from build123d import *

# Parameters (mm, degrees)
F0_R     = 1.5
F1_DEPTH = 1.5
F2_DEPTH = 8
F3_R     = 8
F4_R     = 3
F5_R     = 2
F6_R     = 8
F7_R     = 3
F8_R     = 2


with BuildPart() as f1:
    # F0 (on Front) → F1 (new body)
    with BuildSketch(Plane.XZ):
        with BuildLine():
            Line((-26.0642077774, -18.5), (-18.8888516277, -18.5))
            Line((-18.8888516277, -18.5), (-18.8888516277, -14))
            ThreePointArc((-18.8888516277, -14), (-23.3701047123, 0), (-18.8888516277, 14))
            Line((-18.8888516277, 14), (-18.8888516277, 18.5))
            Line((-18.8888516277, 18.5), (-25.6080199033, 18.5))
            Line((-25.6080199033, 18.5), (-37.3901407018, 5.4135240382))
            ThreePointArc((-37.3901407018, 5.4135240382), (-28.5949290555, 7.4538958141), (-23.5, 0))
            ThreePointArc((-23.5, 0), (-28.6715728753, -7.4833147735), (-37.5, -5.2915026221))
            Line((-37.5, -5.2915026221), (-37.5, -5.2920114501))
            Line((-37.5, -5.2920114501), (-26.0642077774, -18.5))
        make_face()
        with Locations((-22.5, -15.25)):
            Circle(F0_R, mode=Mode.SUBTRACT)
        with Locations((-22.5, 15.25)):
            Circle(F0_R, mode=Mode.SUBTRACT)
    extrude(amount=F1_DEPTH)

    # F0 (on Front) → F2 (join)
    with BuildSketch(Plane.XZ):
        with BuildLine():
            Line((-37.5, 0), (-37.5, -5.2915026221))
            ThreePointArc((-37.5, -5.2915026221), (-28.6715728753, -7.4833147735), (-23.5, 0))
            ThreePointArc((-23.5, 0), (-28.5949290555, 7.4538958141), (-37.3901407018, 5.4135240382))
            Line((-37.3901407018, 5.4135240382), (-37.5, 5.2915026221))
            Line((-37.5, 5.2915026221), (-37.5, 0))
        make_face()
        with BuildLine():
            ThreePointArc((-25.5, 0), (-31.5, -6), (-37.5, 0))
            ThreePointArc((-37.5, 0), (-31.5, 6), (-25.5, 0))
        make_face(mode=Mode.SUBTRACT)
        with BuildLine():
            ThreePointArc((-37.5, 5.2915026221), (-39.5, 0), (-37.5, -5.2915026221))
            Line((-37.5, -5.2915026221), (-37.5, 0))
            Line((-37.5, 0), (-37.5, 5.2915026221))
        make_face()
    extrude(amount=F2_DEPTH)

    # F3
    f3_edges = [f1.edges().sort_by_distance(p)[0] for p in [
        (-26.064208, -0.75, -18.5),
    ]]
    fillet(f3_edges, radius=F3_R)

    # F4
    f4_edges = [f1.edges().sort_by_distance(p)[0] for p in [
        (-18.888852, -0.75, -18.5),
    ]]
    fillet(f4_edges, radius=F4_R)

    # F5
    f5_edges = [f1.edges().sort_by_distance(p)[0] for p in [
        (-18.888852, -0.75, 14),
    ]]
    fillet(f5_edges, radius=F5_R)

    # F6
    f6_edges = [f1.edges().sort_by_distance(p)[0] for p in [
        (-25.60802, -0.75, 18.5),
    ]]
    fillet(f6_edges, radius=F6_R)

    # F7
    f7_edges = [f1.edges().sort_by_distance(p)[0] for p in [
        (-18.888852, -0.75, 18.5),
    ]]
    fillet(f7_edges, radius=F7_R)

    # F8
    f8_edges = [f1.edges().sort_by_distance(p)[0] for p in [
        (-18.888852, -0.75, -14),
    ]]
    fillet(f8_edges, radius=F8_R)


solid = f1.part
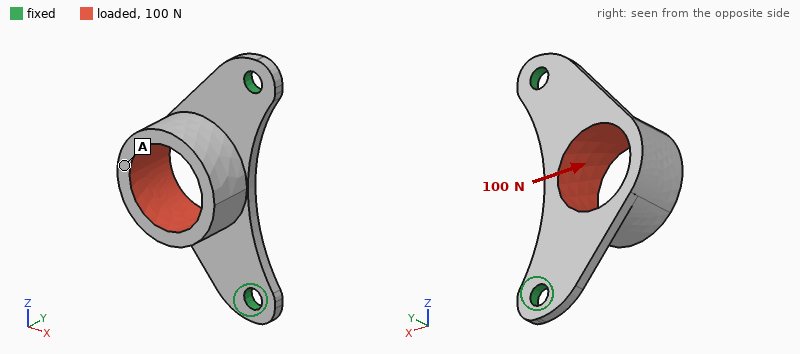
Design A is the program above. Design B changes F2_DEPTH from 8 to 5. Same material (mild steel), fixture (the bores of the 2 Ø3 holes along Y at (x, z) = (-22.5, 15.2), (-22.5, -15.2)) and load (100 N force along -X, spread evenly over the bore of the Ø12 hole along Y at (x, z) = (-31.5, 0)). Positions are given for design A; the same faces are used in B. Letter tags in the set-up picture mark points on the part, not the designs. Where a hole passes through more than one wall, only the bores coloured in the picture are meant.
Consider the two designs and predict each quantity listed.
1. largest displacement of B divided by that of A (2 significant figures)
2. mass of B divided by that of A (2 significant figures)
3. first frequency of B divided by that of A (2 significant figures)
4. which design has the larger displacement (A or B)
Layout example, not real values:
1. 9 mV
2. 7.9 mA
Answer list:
1. 0.55
2. 0.75
3. 1.3
4. A
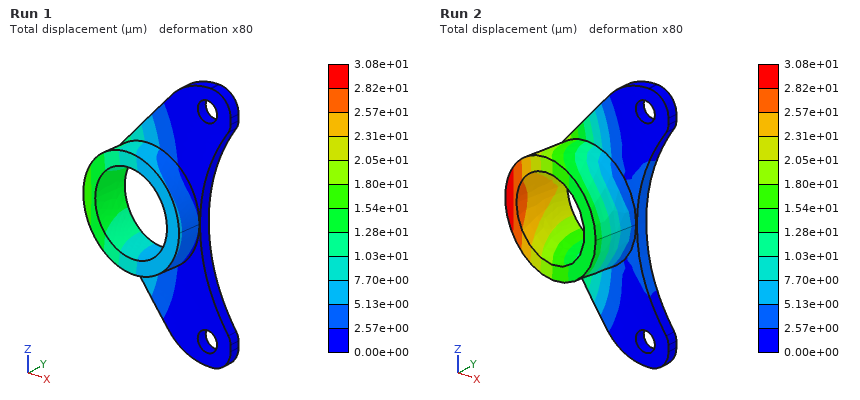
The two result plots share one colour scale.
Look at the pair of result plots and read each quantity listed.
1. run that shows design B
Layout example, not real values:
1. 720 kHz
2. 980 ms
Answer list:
1. Run 1
